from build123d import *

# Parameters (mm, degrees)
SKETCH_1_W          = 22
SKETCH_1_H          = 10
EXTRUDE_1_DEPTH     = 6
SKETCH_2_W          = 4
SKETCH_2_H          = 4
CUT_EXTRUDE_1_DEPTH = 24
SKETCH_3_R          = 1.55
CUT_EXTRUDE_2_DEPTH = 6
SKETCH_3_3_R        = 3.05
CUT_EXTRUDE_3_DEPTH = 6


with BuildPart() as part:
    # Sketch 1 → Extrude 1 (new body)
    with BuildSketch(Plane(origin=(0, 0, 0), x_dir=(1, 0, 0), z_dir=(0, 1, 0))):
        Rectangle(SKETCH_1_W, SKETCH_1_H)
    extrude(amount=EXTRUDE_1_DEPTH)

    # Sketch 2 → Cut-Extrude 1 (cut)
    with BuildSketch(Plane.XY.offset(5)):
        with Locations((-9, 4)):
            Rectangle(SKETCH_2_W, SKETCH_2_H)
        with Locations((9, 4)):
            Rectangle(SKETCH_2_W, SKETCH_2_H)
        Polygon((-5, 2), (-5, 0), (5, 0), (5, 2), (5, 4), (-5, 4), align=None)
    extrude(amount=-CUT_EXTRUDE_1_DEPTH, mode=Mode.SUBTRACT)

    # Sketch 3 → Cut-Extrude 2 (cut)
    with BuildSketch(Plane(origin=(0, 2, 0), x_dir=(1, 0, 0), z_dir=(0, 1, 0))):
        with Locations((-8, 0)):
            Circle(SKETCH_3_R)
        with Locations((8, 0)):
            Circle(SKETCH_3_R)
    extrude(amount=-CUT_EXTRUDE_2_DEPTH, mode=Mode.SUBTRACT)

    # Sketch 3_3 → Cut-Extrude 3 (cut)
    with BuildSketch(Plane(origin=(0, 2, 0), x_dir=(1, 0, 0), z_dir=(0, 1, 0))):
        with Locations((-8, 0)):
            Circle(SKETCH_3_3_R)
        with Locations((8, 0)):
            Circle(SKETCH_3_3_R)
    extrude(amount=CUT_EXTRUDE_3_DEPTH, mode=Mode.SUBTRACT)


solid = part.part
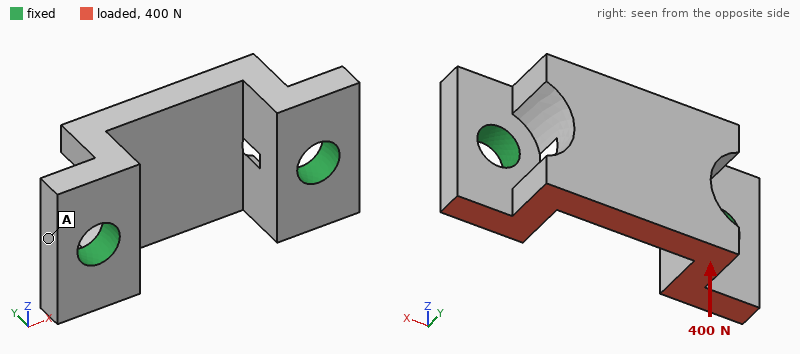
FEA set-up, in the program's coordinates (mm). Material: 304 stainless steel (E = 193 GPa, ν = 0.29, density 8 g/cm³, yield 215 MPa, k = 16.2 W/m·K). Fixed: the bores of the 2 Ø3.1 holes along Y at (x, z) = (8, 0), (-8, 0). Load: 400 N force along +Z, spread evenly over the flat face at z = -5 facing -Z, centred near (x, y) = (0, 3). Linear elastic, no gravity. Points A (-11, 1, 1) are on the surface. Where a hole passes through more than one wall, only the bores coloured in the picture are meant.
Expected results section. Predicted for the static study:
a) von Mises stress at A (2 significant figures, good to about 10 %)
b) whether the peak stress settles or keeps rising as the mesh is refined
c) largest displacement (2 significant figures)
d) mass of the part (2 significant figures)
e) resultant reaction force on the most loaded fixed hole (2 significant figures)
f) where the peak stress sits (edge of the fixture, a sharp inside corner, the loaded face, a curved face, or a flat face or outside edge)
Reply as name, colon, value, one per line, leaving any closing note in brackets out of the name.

von Mises stress at A: 14 MPa
whether the peak stress settles or keeps rising as the mesh is refined: keeps rising
largest displacement: 4.2 µm
mass of the part: 4.0 g
resultant reaction force on the most loaded fixed hole: 200 N
where the peak stress sits: a sharp inside corner
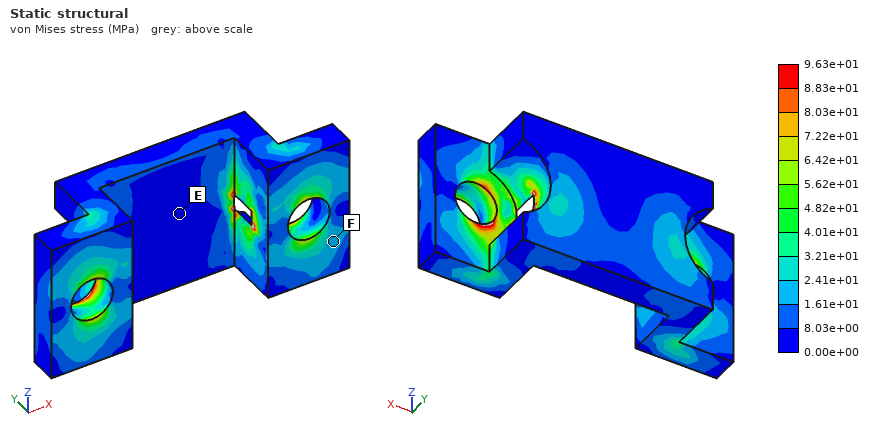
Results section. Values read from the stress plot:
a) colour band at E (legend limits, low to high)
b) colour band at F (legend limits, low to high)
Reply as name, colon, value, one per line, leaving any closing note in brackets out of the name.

colour band at E: 0.00e+00 to 8.03e+00 MPa
colour band at F: 1.61e+01 to 2.41e+01 MPa
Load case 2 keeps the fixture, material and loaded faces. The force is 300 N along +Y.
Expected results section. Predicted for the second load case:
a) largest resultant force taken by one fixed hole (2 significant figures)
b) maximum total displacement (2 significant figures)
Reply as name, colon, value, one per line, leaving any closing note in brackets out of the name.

largest resultant force taken by one fixed hole: 150 N
maximum total displacement: 6.6 µm
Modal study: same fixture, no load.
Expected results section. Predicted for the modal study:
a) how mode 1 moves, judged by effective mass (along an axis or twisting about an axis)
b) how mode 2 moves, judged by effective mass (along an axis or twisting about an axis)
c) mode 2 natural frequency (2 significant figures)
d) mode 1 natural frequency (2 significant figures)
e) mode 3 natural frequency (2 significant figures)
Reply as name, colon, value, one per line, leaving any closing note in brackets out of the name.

how mode 1 moves, judged by effective mass: along Z
how mode 2 moves, judged by effective mass: along X
mode 2 natural frequency: 34 kHz
mode 1 natural frequency: 27 kHz
mode 3 natural frequency: 41 kHz
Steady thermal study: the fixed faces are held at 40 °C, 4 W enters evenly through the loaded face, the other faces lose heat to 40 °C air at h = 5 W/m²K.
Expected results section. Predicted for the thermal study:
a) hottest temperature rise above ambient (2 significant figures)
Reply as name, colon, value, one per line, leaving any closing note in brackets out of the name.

hottest temperature rise above ambient: 52 K
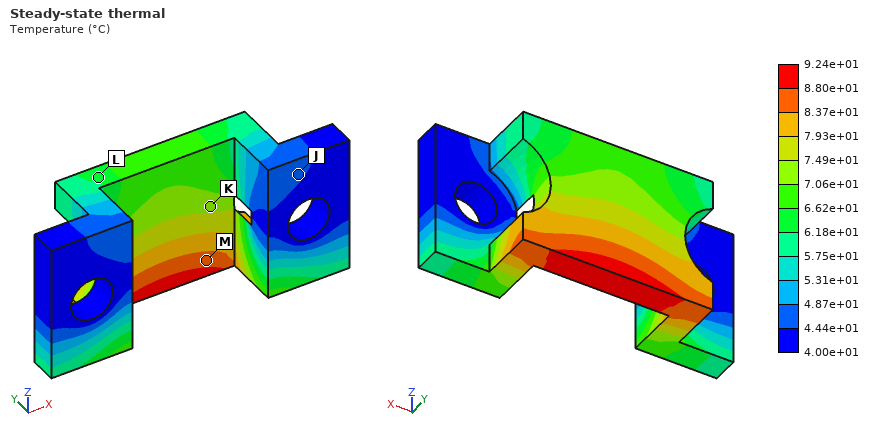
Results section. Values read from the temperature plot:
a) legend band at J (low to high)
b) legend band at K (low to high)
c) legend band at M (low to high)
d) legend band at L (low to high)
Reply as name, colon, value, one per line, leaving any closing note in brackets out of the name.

legend band at J: 4.44e+01 to 4.87e+01 °C
legend band at K: 7.06e+01 to 7.49e+01 °C
legend band at M: 8.37e+01 to 8.80e+01 °C
legend band at L: 6.18e+01 to 6.62e+01 °C
